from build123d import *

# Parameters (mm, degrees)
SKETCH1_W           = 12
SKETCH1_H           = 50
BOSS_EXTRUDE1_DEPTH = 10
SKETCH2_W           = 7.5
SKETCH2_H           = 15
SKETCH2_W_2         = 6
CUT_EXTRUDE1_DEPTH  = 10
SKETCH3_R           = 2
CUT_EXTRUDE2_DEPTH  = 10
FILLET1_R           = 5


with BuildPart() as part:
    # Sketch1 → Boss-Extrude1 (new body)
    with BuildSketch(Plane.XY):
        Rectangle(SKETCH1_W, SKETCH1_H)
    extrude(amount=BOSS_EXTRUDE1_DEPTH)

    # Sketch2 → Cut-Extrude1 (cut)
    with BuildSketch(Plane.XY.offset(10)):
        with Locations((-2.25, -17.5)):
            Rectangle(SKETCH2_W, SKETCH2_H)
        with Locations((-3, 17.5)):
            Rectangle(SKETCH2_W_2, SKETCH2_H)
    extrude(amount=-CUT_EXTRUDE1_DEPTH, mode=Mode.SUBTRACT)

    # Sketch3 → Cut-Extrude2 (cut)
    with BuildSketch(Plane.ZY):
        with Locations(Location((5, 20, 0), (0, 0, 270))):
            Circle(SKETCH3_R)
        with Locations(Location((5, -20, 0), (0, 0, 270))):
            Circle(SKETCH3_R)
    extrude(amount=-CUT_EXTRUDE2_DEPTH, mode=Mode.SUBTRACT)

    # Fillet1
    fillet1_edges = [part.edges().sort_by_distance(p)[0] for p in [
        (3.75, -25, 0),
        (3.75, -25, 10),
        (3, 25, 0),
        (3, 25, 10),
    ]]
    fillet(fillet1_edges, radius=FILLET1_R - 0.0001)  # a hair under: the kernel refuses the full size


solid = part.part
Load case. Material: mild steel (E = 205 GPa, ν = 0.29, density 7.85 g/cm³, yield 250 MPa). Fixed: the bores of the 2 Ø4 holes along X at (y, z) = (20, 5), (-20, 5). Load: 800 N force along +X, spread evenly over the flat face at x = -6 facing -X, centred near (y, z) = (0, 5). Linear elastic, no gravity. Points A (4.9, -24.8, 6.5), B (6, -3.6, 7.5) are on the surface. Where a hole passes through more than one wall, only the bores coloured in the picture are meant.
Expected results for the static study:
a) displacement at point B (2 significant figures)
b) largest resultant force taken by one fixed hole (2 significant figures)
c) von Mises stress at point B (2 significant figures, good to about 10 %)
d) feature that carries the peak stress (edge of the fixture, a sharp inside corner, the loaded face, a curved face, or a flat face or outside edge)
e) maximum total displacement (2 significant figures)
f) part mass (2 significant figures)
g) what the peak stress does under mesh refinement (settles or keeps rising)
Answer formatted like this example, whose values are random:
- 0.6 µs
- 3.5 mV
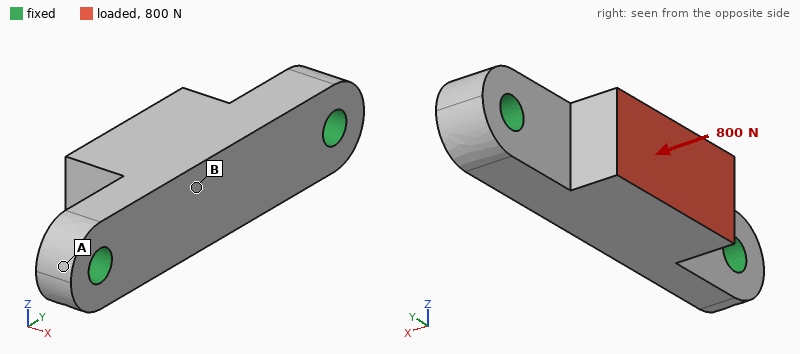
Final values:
- 4.1 µm
- 450 N
- 14 MPa
- edge of the fixture
- 4.3 µm
- 29 g
- keeps rising
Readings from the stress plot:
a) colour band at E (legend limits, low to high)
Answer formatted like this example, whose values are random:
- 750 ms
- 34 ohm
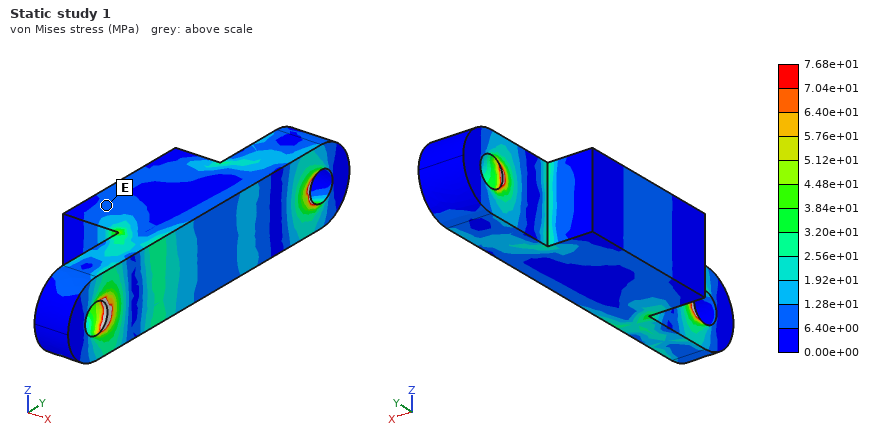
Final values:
- 6.40e+00 to 1.28e+01 MPa
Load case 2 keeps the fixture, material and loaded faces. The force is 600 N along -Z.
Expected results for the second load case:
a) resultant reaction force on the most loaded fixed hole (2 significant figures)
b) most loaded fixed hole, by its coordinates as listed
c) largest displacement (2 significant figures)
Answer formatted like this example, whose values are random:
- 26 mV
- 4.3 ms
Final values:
- 320 N
- (20, 5)
- 15 µm
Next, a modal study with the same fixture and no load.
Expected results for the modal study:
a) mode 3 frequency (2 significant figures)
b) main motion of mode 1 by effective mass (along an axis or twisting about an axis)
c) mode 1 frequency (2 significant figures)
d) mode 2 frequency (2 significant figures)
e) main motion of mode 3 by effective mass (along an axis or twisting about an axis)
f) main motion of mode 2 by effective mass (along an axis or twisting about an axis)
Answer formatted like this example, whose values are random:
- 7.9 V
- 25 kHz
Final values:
- 24 kHz
- along Z
- 12 kHz
- 16 kHz
- along Z
- along X
